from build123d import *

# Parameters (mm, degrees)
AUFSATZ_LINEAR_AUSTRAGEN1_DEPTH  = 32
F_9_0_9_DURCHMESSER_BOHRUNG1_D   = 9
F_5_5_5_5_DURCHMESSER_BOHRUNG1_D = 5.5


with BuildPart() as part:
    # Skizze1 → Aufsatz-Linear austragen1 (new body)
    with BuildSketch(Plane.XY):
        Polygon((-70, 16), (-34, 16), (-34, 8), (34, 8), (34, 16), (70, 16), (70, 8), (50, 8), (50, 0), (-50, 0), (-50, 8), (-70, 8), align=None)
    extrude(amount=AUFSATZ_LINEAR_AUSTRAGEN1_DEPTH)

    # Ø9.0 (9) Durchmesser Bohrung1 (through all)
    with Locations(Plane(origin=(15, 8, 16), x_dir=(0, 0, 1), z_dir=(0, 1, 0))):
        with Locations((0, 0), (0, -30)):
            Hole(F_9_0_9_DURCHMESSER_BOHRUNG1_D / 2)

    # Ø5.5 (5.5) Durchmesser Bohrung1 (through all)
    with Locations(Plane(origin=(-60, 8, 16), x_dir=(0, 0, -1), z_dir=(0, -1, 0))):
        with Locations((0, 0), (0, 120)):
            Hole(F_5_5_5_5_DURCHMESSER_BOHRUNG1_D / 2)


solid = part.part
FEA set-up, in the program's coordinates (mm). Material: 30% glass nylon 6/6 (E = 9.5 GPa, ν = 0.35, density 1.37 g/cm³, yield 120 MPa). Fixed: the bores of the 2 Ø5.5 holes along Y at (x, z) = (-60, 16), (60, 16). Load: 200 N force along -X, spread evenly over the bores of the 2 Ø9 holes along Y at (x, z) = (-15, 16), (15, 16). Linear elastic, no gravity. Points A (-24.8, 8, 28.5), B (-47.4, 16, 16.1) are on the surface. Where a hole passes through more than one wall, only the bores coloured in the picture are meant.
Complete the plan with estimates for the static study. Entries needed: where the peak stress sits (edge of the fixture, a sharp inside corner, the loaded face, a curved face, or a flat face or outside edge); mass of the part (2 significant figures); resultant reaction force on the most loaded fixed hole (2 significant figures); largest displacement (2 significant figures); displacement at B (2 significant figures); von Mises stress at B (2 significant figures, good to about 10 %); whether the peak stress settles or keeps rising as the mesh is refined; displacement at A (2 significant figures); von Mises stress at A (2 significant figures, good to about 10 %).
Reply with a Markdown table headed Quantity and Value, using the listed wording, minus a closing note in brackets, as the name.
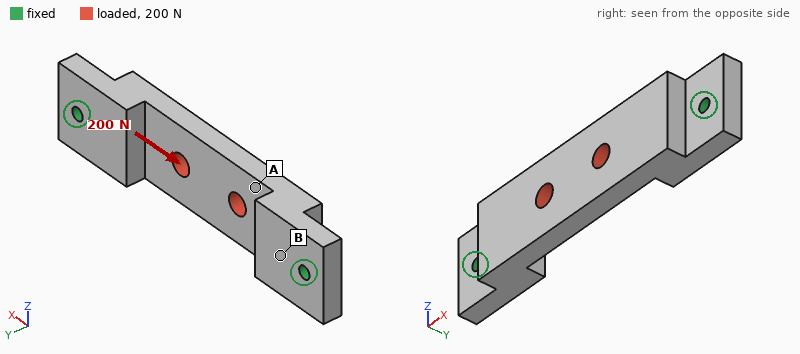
| Quantity | Value |
|---|---|
| where the peak stress sits | edge of the fixture |
| mass of the part | 58 g |
| resultant reaction force on the most loaded fixed hole | 100 N |
| largest displacement | 7.0 µm |
| displacement at B | 1.4 µm |
| von Mises stress at B | 0.25 MPa |
| whether the peak stress settles or keeps rising as the mesh is refined | keeps rising |
| displacement at A | 6.8 µm |
| von Mises stress at A | 1.1 MPa |
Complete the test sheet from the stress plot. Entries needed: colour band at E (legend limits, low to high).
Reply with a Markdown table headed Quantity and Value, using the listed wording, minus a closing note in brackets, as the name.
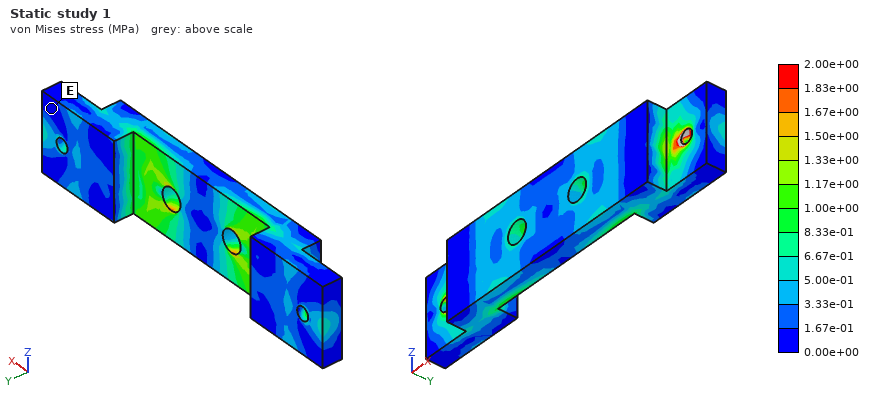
| Quantity | Value |
|---|---|
| colour band at E | 0.00e+00 to 1.67e-01 MPa |
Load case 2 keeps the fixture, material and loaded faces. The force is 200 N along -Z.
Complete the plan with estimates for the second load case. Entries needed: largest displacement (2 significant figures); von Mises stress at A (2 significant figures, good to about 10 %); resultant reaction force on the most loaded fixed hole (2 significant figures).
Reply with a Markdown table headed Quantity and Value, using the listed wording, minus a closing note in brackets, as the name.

| Quantity | Value |
|---|---|
| largest displacement | 36 µm |
| von Mises stress at A | 1.3 MPa |
| resultant reaction force on the most loaded fixed hole | 100 N |
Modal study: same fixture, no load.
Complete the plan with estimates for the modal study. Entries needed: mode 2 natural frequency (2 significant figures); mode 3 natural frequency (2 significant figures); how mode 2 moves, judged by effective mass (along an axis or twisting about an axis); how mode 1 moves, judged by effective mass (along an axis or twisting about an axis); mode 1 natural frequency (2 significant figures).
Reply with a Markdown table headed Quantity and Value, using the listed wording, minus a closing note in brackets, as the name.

| Quantity | Value |
|---|---|
| mode 2 natural frequency | 2400 Hz |
| mode 3 natural frequency | 3200 Hz |
| how mode 2 moves, judged by effective mass | along Z |
| how mode 1 moves, judged by effective mass | along Y |
| mode 1 natural frequency | 2100 Hz |
